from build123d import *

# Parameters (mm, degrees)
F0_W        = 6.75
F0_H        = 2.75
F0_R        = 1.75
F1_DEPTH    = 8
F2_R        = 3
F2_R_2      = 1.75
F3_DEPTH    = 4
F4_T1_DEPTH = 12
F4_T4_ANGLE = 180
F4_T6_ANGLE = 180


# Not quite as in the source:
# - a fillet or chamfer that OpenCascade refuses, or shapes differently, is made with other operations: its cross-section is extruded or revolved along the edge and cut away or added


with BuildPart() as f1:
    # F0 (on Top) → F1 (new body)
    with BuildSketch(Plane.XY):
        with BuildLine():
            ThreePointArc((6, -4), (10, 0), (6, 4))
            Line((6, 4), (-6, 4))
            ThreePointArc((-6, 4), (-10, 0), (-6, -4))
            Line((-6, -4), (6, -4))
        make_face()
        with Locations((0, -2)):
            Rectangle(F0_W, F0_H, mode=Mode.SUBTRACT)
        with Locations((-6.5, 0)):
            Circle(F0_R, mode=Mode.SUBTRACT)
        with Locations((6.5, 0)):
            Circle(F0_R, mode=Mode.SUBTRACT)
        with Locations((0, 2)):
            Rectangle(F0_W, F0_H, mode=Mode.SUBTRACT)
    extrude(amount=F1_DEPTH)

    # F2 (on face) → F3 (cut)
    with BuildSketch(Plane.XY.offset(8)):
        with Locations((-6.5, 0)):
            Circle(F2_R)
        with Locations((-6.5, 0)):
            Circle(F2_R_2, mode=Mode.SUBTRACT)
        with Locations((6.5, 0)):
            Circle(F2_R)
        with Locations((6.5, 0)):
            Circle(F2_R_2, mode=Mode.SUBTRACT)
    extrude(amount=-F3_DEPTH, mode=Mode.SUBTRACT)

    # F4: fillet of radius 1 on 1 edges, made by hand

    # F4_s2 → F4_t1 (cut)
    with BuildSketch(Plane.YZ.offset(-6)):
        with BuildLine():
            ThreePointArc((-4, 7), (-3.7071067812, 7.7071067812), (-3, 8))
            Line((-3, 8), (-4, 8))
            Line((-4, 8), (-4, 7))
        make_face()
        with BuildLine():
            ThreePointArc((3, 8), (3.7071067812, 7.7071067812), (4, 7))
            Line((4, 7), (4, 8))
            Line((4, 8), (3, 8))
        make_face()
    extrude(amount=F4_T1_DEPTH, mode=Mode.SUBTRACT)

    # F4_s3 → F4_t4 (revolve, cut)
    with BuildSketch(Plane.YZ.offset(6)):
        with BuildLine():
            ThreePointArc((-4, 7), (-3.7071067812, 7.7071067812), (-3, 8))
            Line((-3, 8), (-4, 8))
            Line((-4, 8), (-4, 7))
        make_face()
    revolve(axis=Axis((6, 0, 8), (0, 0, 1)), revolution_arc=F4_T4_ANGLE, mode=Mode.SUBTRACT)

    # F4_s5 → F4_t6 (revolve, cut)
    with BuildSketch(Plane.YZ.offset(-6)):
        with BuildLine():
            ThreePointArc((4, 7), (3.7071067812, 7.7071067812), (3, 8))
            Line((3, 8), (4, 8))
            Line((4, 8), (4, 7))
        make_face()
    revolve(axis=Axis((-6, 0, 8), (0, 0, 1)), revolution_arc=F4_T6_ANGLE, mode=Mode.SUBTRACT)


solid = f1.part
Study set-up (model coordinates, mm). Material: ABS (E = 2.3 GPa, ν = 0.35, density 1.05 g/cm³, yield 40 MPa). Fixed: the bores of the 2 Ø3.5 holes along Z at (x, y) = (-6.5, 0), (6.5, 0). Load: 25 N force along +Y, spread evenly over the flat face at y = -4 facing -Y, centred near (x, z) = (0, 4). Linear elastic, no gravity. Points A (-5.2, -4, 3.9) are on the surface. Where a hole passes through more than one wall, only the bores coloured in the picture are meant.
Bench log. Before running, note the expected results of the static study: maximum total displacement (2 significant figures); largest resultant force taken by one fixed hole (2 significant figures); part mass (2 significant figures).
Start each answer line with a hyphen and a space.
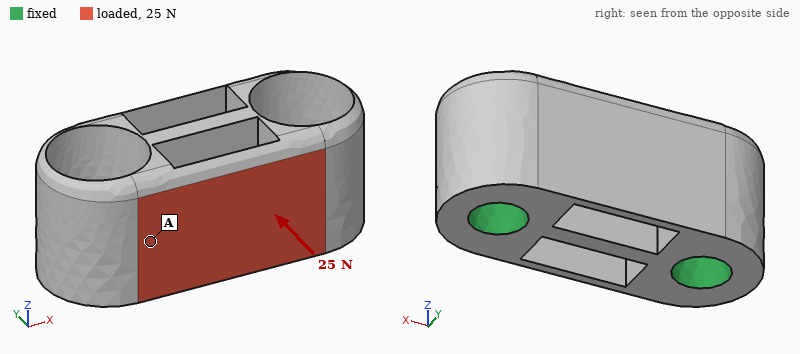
- 54 µm
- 13 N
- 0.59 g
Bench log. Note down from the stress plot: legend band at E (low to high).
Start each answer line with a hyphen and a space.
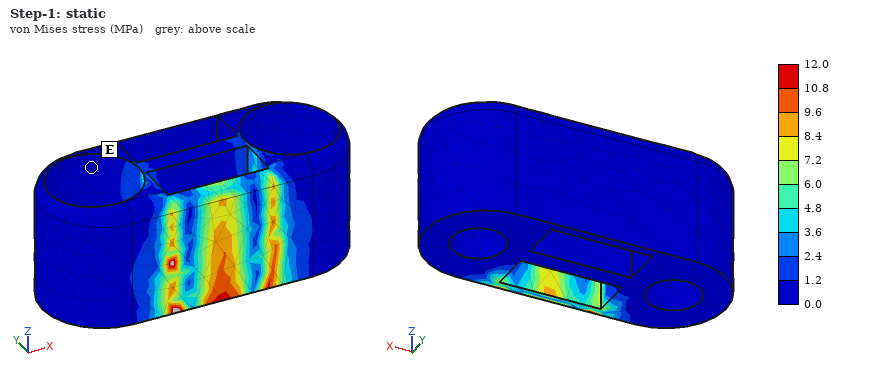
- 0.0 to 1.2 MPa
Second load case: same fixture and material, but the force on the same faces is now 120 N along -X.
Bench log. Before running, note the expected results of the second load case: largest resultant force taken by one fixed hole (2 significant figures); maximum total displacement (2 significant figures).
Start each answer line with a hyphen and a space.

- 61 N
- 29 µm
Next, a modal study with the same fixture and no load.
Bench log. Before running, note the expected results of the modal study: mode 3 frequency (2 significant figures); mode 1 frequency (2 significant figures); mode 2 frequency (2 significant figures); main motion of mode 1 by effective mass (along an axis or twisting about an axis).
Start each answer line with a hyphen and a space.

- 19 kHz
- 15 kHz
- 17 kHz
- along Y
